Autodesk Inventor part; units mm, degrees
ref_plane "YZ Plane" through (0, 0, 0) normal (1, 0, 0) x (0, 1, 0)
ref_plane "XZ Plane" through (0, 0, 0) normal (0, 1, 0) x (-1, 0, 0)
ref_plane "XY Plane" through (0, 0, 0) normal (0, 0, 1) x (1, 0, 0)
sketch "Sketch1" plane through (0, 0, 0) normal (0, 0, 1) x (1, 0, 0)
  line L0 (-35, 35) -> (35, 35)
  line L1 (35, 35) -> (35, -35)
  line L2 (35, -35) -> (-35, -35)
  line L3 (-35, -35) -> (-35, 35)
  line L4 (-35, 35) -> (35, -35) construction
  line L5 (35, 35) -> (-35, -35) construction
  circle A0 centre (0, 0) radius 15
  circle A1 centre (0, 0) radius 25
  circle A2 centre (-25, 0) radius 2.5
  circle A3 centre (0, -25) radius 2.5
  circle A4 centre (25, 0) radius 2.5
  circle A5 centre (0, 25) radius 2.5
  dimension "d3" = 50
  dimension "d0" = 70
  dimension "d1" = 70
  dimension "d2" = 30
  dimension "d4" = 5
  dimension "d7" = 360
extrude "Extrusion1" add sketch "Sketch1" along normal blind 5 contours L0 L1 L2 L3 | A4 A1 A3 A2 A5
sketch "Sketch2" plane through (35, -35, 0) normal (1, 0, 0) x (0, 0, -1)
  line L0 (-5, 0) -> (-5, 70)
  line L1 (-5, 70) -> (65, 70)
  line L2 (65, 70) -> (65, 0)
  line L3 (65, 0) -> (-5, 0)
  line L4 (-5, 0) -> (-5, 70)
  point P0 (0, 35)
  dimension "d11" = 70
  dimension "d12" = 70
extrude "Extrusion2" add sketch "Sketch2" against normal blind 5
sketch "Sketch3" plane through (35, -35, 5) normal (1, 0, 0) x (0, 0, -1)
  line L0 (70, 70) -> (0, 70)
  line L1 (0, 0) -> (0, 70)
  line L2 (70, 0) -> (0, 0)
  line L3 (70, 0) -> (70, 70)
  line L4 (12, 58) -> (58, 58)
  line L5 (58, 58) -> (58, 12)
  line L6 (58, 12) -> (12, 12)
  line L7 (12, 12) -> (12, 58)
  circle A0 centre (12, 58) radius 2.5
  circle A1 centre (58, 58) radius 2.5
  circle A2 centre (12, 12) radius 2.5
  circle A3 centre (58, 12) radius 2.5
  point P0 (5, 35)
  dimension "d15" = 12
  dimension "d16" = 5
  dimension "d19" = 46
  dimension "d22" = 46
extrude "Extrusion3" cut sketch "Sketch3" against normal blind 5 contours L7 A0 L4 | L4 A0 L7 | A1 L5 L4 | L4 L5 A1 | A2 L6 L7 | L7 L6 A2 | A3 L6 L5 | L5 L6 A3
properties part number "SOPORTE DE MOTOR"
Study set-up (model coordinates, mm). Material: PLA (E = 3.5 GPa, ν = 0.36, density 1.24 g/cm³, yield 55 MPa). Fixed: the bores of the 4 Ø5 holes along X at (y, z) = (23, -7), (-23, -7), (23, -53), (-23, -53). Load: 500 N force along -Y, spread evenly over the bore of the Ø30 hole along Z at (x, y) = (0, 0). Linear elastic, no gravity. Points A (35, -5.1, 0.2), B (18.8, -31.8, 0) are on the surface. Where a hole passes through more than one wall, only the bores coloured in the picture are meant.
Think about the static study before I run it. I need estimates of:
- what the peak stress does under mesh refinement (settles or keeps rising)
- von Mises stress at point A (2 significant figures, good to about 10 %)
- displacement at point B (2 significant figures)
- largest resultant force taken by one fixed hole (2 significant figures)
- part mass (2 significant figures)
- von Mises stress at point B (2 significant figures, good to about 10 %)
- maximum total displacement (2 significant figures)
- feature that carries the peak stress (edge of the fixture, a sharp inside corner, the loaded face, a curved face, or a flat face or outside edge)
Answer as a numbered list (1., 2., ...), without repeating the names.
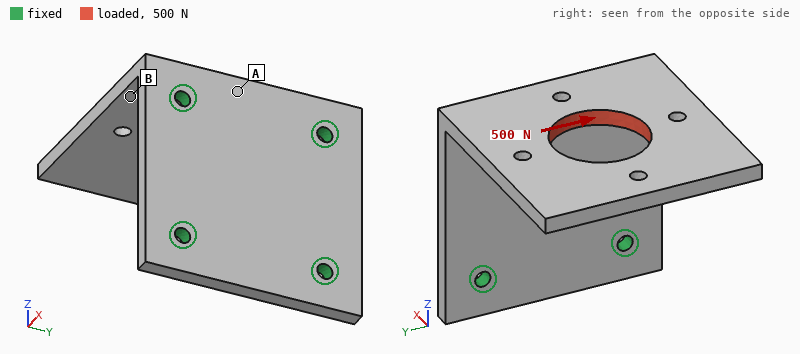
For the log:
1. keeps rising
2. 2.5 MPa
3. 0.21 mm
4. 420 N
5. 53 g
6. 6.1 MPa
7. 0.57 mm
8. edge of the fixture
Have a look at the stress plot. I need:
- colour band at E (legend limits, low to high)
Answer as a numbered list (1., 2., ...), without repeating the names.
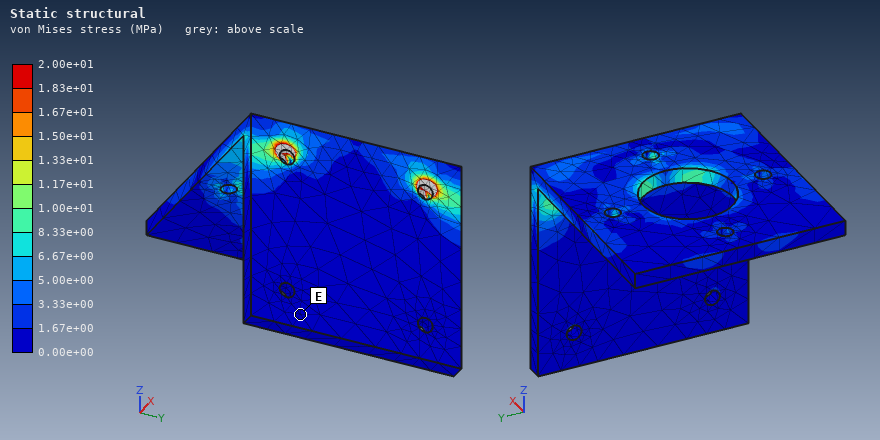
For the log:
1. 0.00e+00 to 1.67e+00 MPa
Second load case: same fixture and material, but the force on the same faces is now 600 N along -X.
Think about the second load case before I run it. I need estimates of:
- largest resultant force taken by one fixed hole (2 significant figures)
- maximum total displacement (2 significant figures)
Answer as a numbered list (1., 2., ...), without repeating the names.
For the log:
1. 320 N
2. 0.87 mm
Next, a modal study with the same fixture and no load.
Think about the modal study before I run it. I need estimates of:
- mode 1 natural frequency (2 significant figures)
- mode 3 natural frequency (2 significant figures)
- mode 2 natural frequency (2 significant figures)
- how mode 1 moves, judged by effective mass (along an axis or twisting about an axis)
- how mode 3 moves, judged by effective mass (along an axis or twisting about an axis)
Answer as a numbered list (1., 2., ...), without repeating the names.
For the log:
1. 240 Hz
2. 1200 Hz
3. 570 Hz
4. along Z
5. along Y
